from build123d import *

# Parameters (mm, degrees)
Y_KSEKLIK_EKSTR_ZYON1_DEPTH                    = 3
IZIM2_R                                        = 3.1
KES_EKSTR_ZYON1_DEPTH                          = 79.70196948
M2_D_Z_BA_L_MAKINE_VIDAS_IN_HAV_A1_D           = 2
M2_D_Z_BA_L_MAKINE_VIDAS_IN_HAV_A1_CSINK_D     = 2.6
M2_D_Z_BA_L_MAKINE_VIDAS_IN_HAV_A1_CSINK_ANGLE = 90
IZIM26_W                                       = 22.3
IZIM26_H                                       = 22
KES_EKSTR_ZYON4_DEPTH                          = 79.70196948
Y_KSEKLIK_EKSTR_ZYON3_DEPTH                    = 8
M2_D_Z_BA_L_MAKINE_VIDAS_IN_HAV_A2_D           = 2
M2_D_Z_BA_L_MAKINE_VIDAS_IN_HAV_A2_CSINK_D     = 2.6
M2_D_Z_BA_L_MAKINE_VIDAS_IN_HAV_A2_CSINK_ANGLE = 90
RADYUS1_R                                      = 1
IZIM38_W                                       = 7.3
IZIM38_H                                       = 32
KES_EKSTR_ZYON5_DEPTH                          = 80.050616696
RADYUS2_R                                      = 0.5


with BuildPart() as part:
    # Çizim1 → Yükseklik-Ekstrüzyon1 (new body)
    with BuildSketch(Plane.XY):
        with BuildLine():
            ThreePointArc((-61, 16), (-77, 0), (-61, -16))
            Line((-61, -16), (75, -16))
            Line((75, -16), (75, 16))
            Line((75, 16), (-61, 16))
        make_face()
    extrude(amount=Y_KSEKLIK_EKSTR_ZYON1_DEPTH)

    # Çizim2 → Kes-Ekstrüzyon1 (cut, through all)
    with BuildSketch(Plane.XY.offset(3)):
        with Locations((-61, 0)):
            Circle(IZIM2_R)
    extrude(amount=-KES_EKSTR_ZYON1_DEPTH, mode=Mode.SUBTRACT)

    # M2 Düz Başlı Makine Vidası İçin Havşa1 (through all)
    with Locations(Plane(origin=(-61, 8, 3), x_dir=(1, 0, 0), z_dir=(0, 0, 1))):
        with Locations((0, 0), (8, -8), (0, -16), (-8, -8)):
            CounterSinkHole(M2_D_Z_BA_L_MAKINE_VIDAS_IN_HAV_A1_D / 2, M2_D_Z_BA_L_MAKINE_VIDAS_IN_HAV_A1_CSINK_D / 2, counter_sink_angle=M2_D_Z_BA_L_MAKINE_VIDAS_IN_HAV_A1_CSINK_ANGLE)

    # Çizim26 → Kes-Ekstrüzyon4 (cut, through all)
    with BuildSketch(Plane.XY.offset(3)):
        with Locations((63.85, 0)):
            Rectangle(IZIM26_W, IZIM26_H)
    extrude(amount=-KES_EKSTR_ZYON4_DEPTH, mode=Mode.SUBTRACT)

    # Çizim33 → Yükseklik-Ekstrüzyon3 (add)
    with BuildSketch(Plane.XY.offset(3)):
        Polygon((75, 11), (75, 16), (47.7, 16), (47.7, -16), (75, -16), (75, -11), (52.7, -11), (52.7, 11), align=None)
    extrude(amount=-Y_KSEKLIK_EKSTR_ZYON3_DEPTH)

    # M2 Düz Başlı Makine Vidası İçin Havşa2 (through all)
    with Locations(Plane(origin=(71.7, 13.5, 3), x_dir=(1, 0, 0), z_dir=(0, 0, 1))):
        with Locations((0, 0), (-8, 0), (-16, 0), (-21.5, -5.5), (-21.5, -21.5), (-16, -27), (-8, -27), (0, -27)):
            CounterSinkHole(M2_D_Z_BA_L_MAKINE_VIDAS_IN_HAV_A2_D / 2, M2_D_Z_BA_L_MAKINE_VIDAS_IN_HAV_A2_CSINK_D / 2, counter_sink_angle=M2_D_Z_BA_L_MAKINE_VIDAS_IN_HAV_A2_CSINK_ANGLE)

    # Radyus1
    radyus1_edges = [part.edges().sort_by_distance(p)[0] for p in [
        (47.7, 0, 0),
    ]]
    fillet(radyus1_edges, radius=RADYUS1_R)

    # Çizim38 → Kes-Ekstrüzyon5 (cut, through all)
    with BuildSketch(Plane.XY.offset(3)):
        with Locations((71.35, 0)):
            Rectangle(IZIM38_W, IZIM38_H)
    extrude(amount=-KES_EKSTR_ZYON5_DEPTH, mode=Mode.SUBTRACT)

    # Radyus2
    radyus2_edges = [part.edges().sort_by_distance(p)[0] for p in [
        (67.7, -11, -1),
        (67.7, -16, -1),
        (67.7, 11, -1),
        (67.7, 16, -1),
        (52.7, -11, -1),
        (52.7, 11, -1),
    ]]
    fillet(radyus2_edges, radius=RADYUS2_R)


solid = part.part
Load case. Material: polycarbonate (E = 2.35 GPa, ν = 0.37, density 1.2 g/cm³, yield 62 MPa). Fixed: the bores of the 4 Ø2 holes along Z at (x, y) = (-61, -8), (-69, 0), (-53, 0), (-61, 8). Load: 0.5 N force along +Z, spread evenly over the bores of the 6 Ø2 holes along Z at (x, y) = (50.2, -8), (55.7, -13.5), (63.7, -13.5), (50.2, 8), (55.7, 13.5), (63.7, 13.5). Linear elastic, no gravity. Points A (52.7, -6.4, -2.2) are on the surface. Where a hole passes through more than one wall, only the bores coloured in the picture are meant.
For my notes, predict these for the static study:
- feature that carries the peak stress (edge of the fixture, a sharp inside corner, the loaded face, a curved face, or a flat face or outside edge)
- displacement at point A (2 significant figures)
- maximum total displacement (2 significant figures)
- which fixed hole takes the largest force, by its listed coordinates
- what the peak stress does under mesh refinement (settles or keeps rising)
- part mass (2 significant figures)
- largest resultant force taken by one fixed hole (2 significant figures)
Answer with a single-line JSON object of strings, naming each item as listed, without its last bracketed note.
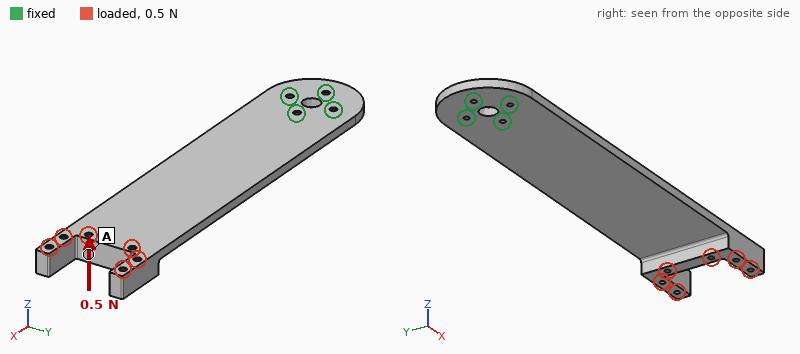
{"feature that carries the peak stress": "edge of the fixture", "displacement at point A": "1.2 mm", "maximum total displacement": "1.5 mm", "which fixed hole takes the largest force, by its listed coordinates": "(-53, 0)", "what the peak stress does under mesh refinement": "keeps rising", "part mass": "17 g", "largest resultant force taken by one fixed hole": "4.6 N"}
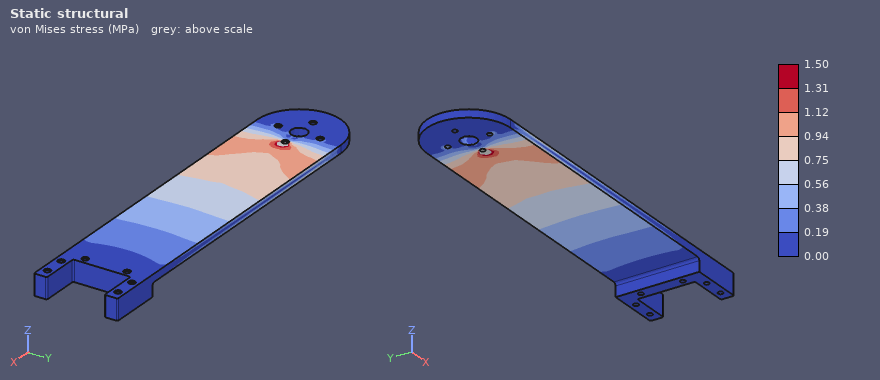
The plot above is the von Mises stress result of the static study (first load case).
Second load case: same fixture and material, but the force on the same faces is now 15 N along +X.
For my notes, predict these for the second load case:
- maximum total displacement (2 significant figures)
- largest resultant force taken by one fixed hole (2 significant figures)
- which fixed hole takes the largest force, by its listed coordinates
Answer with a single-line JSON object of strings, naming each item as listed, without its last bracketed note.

{"maximum total displacement": "1.7 mm", "largest resultant force taken by one fixed hole": "7.2 N", "which fixed hole takes the largest force, by its listed coordinates": "(-53, 0)"}
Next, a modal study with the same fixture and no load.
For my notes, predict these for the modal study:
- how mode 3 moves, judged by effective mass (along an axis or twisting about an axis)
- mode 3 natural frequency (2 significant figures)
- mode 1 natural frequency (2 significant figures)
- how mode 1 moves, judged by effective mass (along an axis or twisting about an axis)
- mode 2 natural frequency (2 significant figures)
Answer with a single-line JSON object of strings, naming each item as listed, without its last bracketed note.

{"how mode 3 moves, judged by effective mass": "along Z", "mode 3 natural frequency": "290 Hz", "mode 1 natural frequency": "45 Hz", "how mode 1 moves, judged by effective mass": "along Z", "mode 2 natural frequency": "280 Hz"}
